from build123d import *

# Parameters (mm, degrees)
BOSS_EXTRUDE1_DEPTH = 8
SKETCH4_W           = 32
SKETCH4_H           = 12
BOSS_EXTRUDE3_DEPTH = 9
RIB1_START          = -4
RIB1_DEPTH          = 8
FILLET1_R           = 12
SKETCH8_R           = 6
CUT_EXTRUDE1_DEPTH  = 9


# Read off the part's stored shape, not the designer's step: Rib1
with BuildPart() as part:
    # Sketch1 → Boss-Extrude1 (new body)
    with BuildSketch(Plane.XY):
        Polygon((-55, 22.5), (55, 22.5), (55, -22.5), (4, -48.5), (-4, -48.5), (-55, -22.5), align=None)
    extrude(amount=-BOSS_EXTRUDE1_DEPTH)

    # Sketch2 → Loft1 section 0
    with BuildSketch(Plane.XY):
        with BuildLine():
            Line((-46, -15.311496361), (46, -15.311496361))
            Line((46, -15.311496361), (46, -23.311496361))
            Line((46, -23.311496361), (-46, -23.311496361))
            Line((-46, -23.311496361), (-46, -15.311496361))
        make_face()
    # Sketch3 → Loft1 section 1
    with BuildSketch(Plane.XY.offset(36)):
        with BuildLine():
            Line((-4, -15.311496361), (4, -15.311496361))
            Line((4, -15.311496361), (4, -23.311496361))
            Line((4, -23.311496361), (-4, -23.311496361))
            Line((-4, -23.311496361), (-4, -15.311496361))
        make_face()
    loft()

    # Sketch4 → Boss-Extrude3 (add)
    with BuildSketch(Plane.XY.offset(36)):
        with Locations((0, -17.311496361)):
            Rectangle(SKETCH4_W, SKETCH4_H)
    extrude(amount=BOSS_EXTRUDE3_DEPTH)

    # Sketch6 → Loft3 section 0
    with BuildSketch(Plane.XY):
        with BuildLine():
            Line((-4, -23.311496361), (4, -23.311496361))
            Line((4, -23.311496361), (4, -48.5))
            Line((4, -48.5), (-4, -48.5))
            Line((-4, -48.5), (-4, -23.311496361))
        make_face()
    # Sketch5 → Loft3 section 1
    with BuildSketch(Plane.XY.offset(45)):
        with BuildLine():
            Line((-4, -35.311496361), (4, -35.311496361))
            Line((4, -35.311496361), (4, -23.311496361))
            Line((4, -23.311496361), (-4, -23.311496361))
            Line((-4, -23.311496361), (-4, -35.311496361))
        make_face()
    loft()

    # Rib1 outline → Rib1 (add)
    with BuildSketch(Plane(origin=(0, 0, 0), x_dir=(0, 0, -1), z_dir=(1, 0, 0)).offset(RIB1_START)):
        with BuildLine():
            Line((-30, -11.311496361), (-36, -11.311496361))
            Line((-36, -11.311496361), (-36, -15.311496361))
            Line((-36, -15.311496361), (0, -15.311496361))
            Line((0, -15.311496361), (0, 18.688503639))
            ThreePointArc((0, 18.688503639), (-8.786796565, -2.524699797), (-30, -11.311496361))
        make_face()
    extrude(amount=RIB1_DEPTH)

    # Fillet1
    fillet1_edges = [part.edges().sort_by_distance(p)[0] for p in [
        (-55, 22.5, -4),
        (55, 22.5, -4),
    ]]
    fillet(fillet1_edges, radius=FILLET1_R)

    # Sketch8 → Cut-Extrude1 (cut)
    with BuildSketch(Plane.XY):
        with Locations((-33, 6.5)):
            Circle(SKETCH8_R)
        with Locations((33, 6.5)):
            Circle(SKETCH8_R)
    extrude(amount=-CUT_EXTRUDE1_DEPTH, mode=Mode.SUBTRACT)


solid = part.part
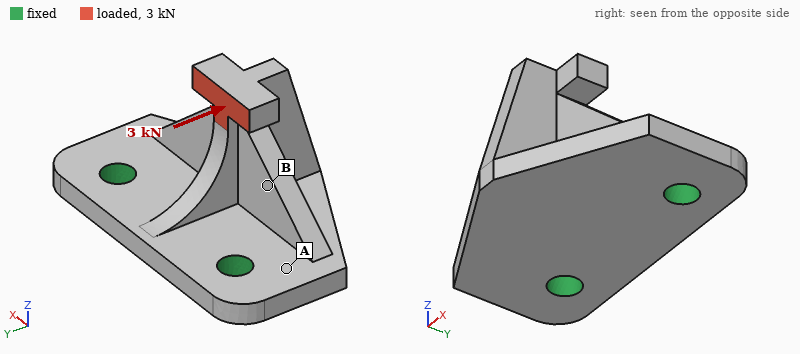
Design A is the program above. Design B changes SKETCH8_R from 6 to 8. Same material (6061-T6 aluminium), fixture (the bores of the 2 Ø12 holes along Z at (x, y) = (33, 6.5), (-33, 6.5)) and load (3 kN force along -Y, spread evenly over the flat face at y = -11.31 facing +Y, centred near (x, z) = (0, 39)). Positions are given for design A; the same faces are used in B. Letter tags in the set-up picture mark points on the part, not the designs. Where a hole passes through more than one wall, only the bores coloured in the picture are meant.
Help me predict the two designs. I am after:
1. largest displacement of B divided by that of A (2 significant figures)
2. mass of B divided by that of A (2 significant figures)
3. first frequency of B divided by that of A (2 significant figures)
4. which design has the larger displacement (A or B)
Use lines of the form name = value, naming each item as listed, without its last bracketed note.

largest displacement of B divided by that of A = 0.85
mass of B divided by that of A = 0.98
first frequency of B divided by that of A = 1.1
which design has the larger displacement = A
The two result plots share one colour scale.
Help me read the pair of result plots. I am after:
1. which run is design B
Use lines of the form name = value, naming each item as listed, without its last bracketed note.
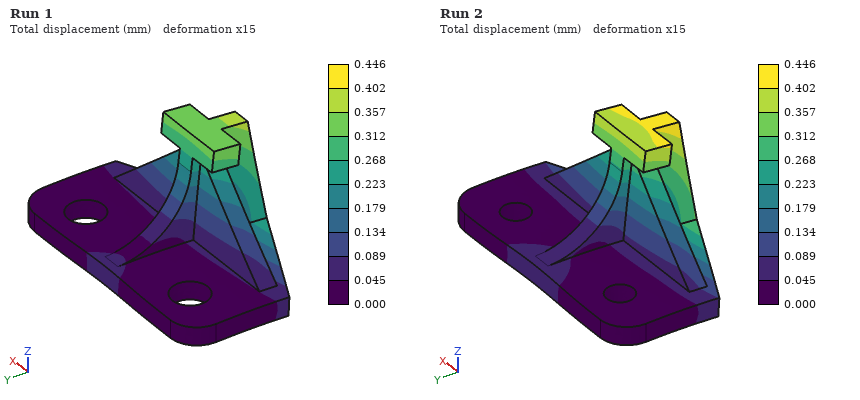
which run is design B = Run 1
